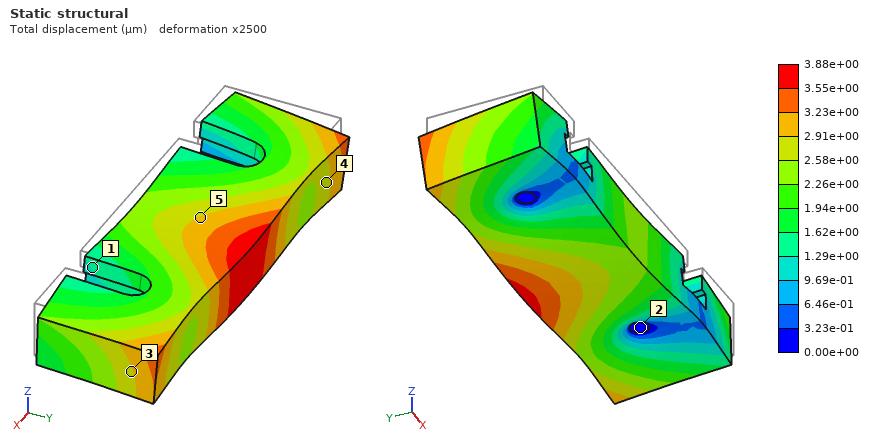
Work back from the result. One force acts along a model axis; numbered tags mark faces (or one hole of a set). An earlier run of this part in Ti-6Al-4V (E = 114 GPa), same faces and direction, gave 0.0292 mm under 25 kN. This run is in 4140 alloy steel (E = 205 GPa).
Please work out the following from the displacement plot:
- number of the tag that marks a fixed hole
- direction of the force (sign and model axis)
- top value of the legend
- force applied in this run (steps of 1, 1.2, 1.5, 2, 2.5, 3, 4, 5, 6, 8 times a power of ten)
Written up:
2
-Z
3.88e+00 µm
6 kN
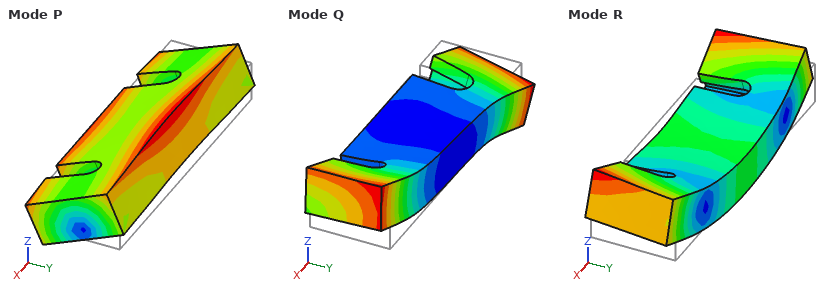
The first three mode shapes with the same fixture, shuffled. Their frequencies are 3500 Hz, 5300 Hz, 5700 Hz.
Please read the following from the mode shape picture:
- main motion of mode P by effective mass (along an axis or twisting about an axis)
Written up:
along Y
